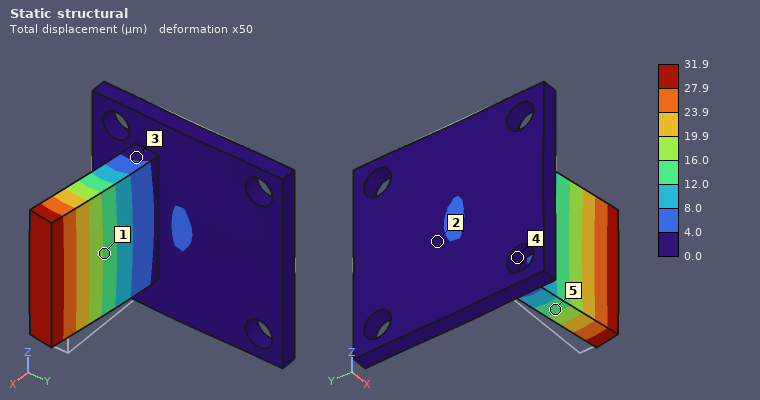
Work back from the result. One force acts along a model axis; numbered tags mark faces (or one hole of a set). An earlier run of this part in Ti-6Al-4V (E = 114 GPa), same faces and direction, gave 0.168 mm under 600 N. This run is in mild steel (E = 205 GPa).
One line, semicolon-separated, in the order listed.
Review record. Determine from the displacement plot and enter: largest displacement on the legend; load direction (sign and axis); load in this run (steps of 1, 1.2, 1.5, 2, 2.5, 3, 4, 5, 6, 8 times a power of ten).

31.9 µm; -Y; 200 N
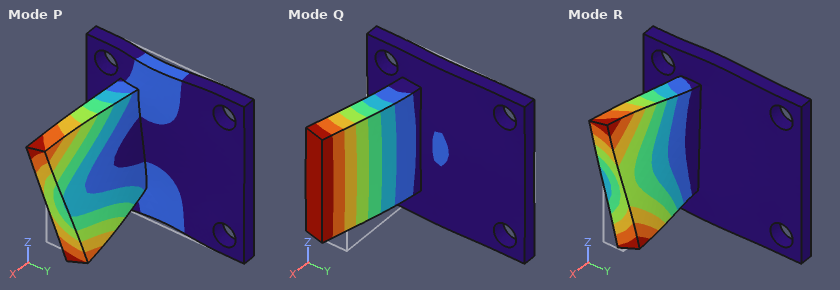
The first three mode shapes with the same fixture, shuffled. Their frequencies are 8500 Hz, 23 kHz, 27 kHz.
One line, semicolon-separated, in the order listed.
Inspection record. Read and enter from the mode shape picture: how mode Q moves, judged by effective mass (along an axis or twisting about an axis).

along Y
